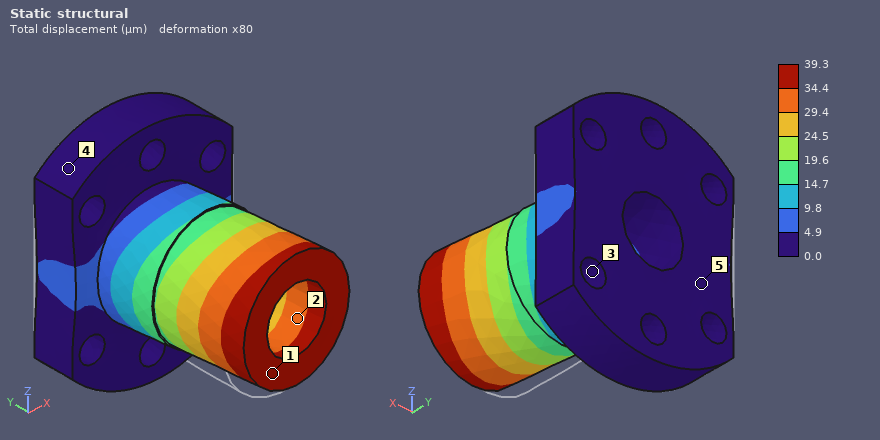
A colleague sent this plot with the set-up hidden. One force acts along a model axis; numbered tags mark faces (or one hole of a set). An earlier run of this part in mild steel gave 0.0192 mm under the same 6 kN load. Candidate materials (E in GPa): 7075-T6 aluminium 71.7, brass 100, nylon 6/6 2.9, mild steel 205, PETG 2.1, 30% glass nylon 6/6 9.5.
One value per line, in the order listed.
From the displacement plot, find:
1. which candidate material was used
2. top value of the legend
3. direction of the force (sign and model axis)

brass
39.3 µm
+X
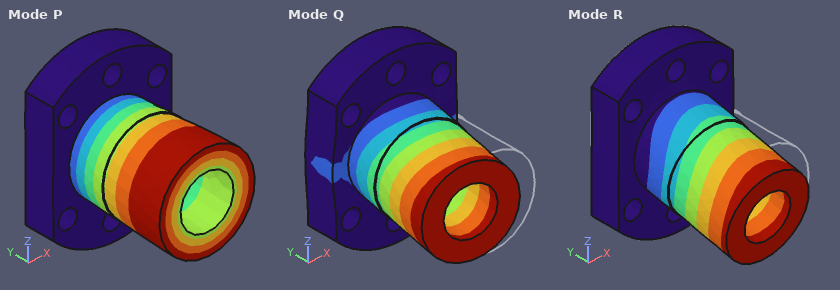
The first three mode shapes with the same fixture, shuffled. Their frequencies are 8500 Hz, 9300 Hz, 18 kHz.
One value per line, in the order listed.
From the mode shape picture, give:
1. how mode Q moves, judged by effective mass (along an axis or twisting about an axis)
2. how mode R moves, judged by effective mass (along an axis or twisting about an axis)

along X
along Z
